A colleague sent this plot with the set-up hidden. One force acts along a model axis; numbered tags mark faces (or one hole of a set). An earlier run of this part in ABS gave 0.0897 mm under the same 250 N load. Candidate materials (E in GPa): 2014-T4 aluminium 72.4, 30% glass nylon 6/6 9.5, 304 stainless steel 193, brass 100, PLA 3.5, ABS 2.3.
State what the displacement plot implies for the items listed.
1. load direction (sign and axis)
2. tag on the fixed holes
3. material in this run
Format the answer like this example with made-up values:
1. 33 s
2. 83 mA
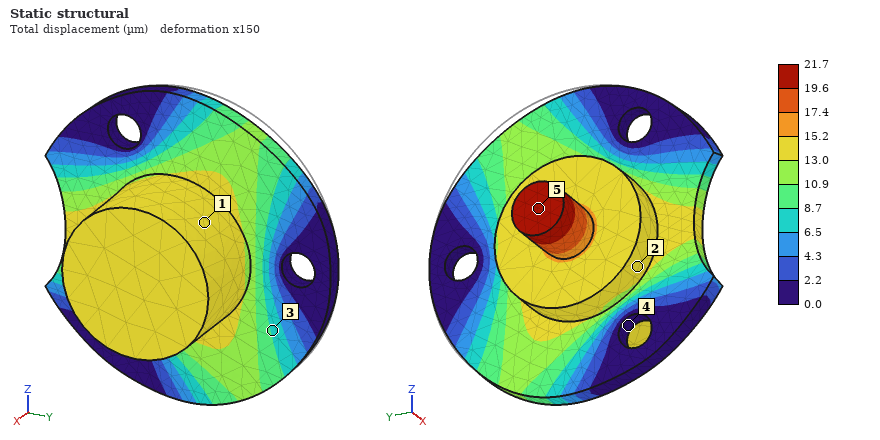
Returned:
1. +X
2. 4
3. 30% glass nylon 6/6
